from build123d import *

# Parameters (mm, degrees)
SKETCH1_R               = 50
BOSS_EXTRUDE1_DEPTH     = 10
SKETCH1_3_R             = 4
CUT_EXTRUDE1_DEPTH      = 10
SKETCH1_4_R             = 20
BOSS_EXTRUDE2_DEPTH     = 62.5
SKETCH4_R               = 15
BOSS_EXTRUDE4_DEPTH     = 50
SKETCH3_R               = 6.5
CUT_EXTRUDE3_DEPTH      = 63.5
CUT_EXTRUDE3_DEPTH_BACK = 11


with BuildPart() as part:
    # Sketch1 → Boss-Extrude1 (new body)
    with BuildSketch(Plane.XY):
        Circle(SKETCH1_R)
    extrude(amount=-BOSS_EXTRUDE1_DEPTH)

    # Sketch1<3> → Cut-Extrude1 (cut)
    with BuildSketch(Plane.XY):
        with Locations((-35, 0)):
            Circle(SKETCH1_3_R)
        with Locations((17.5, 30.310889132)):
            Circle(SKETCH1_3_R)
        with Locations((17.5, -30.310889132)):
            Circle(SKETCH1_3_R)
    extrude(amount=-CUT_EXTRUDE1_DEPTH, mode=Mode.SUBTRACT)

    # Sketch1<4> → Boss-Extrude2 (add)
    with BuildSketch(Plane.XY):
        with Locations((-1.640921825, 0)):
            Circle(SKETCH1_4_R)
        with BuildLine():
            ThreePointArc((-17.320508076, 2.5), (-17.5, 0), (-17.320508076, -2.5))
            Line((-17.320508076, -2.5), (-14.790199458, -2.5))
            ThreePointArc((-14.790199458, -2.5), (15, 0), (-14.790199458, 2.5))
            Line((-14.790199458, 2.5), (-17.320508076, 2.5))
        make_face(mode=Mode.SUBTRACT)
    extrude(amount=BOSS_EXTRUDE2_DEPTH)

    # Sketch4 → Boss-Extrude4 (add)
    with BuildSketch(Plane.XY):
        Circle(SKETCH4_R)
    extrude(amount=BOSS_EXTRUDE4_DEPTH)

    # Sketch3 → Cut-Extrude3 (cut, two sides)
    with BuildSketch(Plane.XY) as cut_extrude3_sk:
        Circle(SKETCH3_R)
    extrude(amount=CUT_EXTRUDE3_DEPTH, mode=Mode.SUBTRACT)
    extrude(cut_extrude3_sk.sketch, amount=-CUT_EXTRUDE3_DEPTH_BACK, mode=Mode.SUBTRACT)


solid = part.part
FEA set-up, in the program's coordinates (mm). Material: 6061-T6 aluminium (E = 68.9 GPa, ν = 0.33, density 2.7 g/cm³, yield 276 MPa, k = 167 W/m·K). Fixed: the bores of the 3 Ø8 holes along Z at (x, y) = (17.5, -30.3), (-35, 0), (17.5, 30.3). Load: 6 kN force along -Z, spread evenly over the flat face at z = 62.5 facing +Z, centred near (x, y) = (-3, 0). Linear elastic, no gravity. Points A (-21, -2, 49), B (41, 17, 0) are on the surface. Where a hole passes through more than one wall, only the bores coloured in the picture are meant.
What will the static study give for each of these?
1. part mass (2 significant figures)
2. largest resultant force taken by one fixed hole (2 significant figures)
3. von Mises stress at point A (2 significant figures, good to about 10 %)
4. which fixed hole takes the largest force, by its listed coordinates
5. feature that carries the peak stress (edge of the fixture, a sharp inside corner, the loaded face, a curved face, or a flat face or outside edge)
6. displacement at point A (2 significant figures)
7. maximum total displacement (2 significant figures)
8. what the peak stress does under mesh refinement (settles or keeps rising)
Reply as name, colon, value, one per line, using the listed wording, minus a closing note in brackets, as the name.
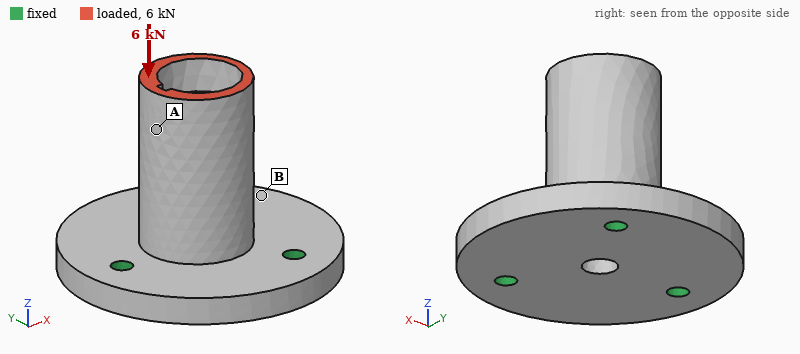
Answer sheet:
part mass: 370 g
largest resultant force taken by one fixed hole: 2.5 kN
von Mises stress at point A: 9.9 MPa
which fixed hole takes the largest force, by its listed coordinates: (-35, 0)
feature that carries the peak stress: edge of the fixture
displacement at point A: 18 µm
maximum total displacement: 20 µm
what the peak stress does under mesh refinement: keeps rising
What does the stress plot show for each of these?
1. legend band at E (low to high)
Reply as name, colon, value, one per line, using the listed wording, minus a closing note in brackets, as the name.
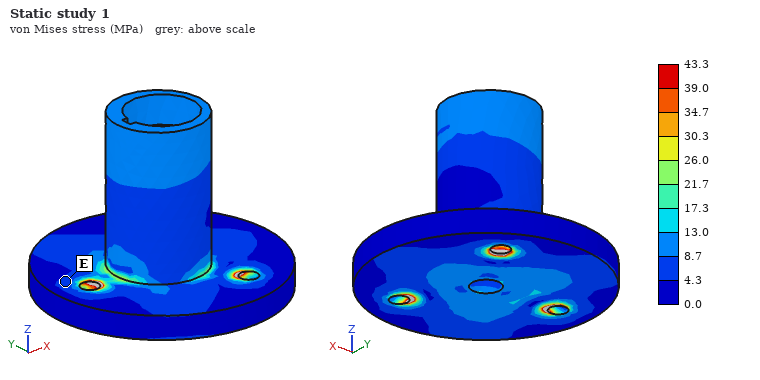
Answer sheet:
legend band at E: 4.3 to 8.7 MPa
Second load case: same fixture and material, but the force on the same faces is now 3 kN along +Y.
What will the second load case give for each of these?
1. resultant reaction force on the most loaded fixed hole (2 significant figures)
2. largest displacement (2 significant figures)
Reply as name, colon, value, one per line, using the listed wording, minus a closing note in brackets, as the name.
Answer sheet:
resultant reaction force on the most loaded fixed hole: 3.6 kN
largest displacement: 0.12 mm
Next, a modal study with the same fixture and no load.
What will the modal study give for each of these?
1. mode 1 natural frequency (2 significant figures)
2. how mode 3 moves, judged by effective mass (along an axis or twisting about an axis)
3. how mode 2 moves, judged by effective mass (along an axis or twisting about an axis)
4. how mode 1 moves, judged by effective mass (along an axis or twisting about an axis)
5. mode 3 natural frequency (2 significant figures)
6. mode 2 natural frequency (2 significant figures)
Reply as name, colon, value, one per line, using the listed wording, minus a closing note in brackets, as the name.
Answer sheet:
mode 1 natural frequency: 3700 Hz
how mode 3 moves, judged by effective mass: along Z
how mode 2 moves, judged by effective mass: along X
how mode 1 moves, judged by effective mass: along Y
mode 3 natural frequency: 7000 Hz
mode 2 natural frequency: 3900 Hz
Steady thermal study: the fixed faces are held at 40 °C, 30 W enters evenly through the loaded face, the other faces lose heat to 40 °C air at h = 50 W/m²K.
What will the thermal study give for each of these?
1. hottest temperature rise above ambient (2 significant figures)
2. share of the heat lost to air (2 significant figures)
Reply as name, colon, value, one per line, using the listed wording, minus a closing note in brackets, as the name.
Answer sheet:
hottest temperature rise above ambient: 15 K
share of the heat lost to air: 20 %
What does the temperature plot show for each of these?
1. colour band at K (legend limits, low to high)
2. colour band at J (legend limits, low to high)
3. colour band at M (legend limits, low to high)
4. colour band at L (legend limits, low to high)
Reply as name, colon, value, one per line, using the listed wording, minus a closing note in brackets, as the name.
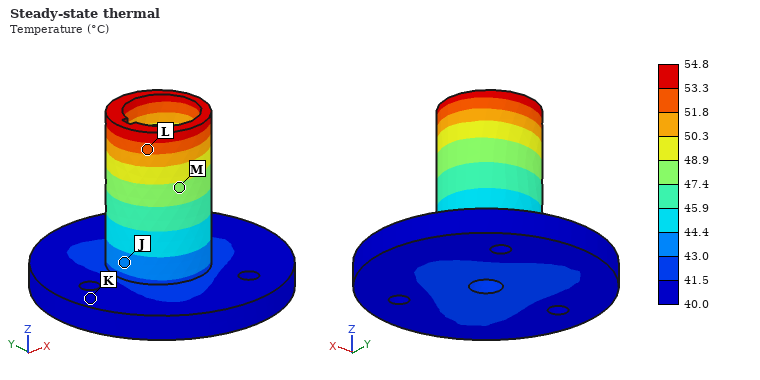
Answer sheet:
colour band at K: 40.0 to 41.5 °C
colour band at J: 43.0 to 44.4 °C
colour band at M: 47.4 to 48.9 °C
colour band at L: 51.8 to 53.3 °C
